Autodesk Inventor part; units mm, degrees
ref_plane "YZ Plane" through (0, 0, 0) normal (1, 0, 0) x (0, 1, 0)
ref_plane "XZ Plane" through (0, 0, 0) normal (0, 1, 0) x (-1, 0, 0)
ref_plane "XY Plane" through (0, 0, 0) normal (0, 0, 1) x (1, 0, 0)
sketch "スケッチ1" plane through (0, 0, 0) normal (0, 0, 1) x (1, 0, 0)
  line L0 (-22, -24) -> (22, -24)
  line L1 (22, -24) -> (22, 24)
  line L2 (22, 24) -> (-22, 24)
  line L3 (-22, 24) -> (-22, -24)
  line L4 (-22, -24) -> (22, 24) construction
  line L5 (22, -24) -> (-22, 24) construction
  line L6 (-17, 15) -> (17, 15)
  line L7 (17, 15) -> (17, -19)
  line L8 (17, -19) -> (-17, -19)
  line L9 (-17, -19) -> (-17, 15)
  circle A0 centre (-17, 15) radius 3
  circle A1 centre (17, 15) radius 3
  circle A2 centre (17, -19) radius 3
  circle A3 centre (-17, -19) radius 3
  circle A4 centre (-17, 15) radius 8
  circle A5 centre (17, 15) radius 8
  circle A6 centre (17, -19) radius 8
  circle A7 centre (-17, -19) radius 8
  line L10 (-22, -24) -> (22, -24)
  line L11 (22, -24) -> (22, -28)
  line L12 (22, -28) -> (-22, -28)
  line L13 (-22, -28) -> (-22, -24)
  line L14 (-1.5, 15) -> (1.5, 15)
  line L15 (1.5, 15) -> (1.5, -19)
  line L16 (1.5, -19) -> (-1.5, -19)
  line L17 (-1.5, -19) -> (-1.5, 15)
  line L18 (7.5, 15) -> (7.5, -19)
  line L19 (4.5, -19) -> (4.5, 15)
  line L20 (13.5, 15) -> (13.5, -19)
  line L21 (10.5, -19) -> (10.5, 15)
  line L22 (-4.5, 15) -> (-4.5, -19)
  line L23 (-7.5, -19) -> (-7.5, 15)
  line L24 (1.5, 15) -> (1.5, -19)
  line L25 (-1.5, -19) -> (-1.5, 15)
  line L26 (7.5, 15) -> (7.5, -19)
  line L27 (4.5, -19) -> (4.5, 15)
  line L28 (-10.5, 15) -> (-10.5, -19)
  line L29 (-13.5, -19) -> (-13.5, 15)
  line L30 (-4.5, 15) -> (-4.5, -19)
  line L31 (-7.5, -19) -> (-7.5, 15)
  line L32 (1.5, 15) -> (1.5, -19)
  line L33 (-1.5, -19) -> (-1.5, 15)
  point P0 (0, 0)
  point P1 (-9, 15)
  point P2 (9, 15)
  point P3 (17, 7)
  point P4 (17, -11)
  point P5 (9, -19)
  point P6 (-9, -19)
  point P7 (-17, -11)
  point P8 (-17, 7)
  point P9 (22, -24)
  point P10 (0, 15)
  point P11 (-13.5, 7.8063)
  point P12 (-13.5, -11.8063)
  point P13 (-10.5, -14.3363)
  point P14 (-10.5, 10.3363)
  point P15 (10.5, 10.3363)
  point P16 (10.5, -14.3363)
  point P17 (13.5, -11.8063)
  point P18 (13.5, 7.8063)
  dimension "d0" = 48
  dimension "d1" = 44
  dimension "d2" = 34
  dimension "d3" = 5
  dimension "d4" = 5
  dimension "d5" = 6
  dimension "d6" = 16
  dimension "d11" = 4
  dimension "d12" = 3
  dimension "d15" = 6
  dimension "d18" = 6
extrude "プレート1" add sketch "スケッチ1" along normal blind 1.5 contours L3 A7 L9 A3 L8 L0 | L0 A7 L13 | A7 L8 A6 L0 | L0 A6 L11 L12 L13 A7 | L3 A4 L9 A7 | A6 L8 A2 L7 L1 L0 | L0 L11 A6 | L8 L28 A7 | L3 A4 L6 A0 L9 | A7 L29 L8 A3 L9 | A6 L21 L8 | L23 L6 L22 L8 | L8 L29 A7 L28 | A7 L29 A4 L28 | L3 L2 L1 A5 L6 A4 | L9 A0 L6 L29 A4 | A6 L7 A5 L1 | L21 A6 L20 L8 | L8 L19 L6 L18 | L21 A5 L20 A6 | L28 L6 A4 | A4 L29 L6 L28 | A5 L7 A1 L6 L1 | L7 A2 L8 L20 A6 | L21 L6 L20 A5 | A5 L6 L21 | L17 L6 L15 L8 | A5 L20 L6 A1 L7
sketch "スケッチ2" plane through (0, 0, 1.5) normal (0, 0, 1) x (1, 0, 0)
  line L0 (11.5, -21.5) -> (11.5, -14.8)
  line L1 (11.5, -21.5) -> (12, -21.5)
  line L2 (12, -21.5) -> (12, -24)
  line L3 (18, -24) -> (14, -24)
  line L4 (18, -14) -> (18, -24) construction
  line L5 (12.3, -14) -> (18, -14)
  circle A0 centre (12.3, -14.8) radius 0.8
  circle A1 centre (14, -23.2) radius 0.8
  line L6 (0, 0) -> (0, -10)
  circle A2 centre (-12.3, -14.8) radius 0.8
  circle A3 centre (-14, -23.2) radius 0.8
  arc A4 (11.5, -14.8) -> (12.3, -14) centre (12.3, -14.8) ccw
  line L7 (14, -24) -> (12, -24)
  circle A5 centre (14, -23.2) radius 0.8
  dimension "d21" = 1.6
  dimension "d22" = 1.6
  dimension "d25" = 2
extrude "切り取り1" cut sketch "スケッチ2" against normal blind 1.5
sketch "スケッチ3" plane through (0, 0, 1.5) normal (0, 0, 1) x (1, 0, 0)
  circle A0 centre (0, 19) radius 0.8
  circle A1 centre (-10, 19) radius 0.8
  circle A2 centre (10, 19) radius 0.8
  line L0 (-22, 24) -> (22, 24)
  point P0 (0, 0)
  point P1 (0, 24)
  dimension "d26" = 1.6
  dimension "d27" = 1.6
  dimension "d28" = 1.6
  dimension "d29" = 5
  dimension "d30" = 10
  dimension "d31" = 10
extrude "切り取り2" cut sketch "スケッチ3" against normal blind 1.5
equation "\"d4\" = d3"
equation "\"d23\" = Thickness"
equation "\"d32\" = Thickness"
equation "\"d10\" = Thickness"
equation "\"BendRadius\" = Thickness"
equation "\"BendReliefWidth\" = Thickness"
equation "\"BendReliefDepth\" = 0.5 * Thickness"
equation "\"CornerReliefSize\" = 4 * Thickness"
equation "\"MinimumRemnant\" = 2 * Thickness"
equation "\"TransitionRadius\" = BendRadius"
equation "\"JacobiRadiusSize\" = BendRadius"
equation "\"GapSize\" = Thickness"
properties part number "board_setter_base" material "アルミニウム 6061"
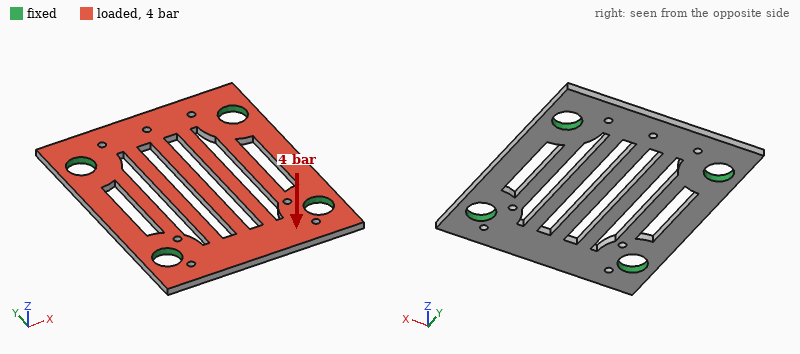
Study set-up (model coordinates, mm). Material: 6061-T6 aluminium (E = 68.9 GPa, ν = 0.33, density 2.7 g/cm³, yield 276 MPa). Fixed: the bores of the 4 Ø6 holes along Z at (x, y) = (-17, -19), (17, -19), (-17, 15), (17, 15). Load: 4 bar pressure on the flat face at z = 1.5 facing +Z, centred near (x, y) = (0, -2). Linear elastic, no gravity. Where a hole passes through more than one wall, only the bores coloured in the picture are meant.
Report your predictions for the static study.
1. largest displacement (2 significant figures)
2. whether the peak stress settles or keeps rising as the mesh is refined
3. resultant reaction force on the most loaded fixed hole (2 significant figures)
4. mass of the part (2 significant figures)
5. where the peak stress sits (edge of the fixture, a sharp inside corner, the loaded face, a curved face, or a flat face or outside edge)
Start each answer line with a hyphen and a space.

- 0.25 mm
- keeps rising
- 160 N
- 6.7 g
- edge of the fixture
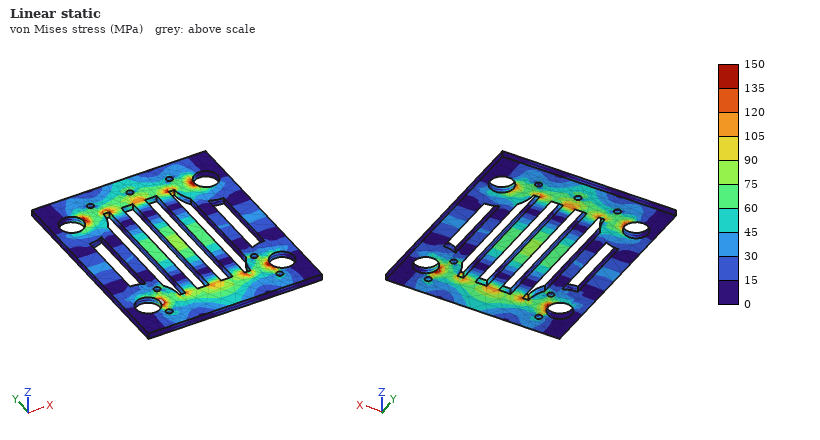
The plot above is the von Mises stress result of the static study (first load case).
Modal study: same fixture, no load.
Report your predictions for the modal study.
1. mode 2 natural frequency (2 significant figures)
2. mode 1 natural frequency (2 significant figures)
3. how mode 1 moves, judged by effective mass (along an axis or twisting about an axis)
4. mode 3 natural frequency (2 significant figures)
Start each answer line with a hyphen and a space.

- 5100 Hz
- 3900 Hz
- along Z
- 5400 Hz
